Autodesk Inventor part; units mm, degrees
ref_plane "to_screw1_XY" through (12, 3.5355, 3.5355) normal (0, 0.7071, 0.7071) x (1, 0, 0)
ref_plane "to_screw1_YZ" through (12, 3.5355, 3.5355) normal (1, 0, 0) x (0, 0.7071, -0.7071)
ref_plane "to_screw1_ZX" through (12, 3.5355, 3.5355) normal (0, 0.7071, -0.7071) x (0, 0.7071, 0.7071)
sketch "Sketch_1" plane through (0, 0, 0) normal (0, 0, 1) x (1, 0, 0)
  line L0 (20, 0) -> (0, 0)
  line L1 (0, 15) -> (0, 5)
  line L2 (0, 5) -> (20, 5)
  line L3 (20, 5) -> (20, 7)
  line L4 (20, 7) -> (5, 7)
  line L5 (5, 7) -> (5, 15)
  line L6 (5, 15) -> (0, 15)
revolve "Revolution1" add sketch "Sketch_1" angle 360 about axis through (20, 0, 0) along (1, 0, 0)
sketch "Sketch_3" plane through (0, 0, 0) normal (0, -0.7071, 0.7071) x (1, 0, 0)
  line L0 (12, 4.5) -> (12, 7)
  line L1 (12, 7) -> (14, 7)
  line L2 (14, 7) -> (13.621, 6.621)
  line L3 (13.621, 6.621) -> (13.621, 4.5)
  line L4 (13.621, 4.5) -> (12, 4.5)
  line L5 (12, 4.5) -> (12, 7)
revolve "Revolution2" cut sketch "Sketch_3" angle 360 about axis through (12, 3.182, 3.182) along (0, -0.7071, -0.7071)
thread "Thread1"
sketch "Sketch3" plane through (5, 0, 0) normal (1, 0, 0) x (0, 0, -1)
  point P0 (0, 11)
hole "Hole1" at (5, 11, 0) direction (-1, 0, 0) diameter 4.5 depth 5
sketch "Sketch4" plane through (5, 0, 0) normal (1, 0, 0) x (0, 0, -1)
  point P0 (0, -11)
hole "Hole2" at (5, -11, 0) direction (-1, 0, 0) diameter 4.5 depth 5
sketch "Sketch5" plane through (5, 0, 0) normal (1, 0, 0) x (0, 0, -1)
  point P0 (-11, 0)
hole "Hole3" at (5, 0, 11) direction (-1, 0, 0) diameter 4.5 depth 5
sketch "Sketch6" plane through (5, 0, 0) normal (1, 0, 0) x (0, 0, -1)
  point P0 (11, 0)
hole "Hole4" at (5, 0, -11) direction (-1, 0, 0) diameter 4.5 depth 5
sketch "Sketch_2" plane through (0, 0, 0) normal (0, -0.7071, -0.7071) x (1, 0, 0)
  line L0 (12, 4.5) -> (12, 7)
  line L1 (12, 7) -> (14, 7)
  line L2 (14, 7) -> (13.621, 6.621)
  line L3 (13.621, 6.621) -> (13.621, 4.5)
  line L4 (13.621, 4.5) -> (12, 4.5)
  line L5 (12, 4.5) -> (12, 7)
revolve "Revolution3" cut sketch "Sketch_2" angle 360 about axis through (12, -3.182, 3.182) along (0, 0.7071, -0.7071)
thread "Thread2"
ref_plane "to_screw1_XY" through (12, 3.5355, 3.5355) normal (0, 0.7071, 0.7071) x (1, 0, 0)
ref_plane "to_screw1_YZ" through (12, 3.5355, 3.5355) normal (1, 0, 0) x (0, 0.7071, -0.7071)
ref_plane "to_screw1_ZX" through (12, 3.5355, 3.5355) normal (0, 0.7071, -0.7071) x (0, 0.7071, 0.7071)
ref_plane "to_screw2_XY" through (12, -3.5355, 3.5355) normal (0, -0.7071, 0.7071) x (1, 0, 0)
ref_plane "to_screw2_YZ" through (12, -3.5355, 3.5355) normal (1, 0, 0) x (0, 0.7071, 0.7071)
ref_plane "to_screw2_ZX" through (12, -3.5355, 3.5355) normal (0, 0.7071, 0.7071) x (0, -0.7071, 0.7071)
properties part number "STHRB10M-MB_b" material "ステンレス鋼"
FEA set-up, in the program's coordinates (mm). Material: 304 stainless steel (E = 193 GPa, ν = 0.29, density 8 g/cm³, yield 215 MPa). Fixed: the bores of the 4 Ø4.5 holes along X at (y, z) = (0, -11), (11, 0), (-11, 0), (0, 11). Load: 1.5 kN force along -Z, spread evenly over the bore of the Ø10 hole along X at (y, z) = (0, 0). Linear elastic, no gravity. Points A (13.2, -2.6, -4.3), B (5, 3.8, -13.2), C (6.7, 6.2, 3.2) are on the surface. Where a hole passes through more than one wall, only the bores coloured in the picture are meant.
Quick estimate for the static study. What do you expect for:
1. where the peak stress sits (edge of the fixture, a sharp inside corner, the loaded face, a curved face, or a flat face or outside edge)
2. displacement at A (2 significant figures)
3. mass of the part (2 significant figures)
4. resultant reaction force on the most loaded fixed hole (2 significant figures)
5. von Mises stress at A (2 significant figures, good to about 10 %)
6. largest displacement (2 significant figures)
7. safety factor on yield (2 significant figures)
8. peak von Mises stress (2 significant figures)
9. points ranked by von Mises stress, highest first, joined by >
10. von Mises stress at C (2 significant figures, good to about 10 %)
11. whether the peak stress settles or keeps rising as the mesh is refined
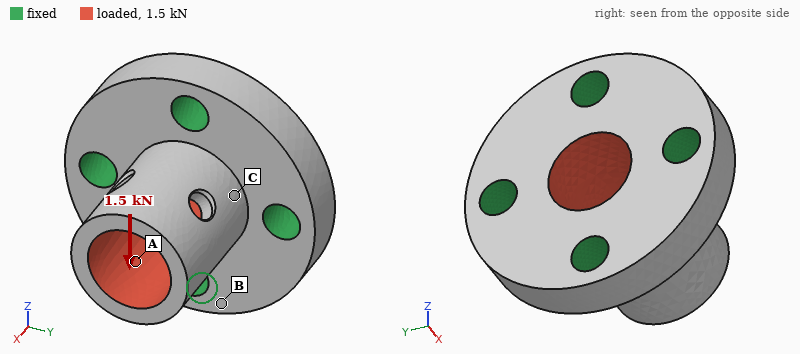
a curved face
4.8 µm
31 g
750 N
20 MPa
7.9 µm
2.8
78 MPa
C > A > B
33 MPa
settles
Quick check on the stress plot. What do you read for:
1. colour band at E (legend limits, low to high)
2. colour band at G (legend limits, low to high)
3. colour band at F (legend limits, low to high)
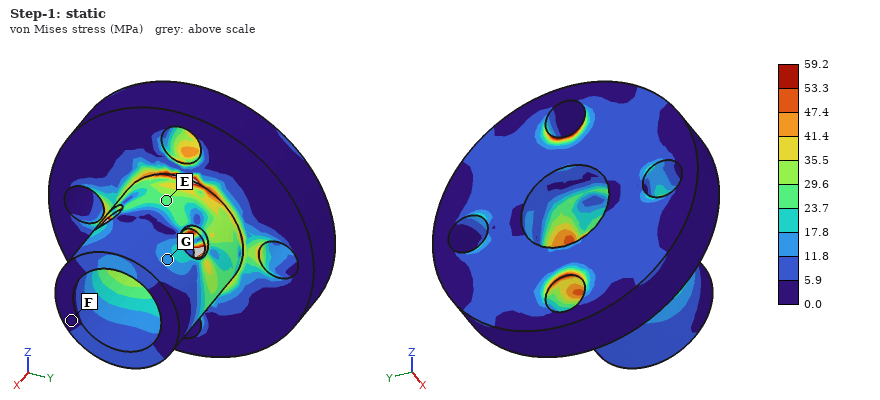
23.7 to 29.6 MPa
11.8 to 17.8 MPa
0.0 to 5.9 MPa
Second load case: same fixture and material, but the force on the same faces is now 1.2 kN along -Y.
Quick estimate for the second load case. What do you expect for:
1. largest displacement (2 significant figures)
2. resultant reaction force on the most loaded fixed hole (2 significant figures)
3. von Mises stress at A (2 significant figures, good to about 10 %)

6.3 µm
590 N
21 MPa
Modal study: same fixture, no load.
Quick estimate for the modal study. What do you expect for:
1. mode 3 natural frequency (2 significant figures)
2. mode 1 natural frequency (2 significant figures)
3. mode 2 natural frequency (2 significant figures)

37 kHz
24 kHz
24 kHz
